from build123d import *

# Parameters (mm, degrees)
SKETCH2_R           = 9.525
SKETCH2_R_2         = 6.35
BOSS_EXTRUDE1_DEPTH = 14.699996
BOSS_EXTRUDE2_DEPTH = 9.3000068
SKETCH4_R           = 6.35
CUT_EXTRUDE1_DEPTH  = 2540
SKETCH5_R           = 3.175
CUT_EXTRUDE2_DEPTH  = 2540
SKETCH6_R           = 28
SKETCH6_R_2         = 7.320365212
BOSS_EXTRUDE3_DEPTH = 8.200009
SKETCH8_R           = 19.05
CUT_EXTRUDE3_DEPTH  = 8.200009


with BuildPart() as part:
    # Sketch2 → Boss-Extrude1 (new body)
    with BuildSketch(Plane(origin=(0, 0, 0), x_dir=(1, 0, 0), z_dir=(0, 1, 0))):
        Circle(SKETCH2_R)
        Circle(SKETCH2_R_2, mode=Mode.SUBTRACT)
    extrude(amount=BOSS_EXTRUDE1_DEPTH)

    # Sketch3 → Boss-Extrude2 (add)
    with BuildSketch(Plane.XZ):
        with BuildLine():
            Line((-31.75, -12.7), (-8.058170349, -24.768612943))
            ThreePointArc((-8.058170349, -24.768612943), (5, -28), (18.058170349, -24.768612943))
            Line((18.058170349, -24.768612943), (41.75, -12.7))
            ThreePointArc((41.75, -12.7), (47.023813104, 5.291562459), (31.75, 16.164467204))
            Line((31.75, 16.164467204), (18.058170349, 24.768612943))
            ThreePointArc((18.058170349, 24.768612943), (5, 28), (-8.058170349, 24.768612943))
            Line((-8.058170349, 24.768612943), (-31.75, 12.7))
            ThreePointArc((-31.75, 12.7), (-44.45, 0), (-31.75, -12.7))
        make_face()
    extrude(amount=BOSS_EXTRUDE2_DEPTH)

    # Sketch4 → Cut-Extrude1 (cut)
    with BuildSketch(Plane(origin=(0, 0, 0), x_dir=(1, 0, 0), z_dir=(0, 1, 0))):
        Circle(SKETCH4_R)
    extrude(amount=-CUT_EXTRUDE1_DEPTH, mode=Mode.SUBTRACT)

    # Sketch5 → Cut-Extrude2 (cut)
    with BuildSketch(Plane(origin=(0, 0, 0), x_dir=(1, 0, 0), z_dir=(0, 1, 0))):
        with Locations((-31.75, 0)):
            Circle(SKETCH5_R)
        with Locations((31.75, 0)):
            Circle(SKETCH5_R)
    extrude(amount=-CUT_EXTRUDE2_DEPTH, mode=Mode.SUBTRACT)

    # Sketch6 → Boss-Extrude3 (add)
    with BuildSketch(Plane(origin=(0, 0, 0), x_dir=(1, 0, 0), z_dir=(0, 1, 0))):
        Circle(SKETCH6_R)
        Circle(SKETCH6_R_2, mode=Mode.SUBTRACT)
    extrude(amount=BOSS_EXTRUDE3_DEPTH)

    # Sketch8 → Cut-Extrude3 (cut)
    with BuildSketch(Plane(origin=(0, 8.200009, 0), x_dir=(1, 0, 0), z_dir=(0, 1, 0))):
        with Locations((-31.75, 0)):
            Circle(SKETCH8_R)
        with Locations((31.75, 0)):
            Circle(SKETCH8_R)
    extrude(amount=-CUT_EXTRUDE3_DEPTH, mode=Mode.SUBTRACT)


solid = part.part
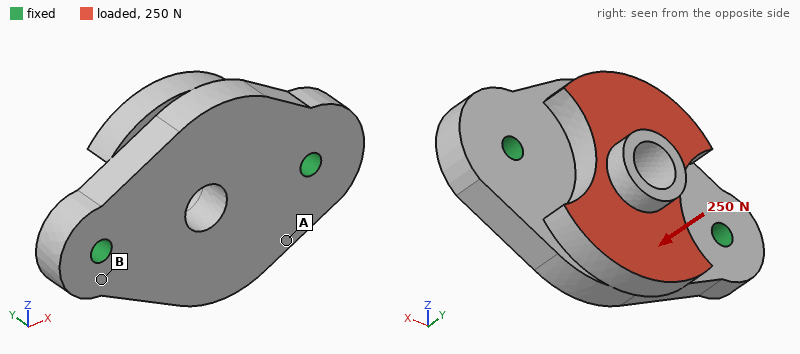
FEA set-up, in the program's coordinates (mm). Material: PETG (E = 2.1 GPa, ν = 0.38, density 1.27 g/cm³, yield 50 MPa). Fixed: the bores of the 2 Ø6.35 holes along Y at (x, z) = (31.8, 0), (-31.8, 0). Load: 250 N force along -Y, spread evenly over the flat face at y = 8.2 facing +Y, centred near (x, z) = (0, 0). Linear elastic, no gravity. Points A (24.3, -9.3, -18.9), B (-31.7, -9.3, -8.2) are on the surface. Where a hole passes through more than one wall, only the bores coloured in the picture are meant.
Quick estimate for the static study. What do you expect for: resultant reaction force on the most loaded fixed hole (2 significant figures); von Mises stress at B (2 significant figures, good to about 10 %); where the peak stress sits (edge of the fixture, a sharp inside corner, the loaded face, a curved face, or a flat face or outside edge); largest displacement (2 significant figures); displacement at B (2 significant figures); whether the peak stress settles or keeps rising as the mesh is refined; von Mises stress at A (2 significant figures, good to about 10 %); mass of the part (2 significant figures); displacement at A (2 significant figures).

140 N
1.2 MPa
edge of the fixture
51 µm
7.9 µm
keeps rising
0.40 MPa
58 g
27 µm
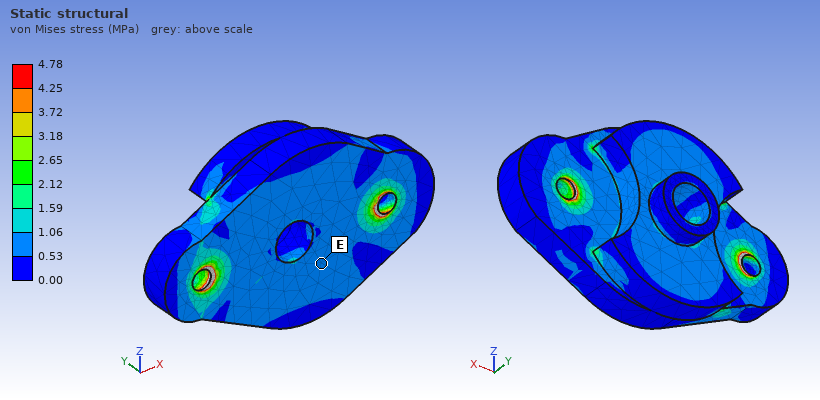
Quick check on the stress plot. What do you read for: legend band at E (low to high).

0.53 to 1.06 MPa
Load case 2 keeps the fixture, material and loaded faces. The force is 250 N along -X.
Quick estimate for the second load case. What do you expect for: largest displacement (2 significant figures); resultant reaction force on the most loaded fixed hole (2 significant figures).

21 µm
140 N
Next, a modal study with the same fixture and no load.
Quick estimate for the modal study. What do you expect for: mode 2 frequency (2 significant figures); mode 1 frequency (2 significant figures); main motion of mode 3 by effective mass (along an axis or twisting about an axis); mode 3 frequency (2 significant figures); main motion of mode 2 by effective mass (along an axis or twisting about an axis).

2000 Hz
1300 Hz
along Z
3600 Hz
along Y
